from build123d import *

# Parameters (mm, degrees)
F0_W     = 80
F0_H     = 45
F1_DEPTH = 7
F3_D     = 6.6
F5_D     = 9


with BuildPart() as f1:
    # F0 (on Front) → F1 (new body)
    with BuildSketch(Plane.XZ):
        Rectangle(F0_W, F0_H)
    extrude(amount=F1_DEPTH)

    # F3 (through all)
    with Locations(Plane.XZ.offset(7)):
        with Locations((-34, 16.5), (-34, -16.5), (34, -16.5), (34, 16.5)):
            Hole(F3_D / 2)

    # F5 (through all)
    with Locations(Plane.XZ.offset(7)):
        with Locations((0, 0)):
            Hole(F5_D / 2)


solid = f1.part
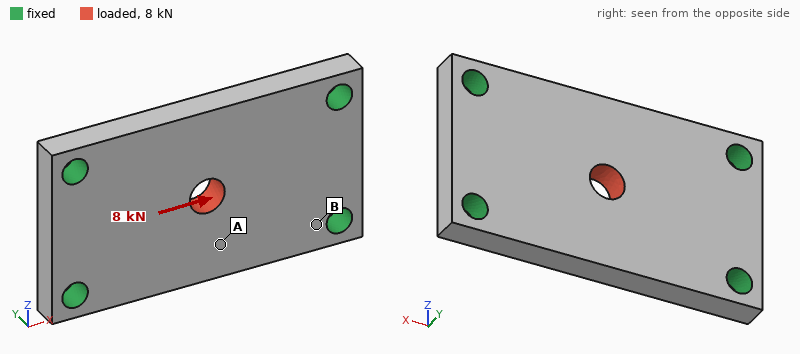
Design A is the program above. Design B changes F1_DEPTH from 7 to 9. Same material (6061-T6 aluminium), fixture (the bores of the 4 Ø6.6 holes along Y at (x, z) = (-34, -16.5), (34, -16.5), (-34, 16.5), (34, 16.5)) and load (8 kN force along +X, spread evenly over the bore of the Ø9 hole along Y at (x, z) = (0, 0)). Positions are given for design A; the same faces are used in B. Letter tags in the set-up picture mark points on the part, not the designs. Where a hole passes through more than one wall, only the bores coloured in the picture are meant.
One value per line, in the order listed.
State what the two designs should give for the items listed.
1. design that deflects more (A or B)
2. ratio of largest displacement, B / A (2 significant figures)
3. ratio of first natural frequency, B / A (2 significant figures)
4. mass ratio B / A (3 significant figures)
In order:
A
0.78
1.2
1.29
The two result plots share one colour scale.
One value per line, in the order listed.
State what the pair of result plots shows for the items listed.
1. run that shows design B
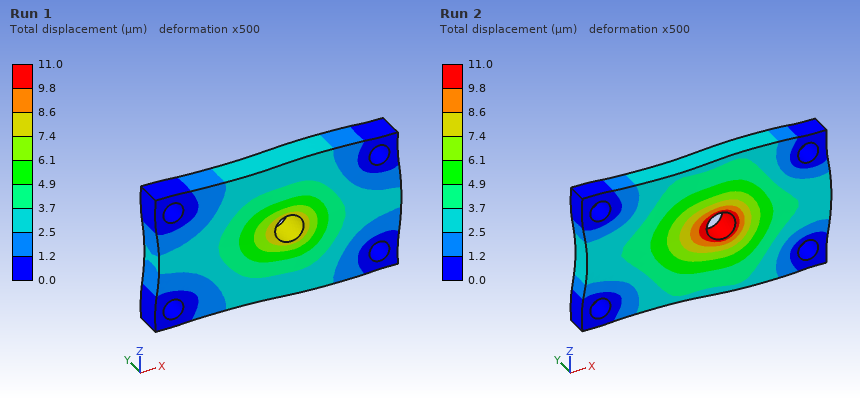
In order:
Run 1
